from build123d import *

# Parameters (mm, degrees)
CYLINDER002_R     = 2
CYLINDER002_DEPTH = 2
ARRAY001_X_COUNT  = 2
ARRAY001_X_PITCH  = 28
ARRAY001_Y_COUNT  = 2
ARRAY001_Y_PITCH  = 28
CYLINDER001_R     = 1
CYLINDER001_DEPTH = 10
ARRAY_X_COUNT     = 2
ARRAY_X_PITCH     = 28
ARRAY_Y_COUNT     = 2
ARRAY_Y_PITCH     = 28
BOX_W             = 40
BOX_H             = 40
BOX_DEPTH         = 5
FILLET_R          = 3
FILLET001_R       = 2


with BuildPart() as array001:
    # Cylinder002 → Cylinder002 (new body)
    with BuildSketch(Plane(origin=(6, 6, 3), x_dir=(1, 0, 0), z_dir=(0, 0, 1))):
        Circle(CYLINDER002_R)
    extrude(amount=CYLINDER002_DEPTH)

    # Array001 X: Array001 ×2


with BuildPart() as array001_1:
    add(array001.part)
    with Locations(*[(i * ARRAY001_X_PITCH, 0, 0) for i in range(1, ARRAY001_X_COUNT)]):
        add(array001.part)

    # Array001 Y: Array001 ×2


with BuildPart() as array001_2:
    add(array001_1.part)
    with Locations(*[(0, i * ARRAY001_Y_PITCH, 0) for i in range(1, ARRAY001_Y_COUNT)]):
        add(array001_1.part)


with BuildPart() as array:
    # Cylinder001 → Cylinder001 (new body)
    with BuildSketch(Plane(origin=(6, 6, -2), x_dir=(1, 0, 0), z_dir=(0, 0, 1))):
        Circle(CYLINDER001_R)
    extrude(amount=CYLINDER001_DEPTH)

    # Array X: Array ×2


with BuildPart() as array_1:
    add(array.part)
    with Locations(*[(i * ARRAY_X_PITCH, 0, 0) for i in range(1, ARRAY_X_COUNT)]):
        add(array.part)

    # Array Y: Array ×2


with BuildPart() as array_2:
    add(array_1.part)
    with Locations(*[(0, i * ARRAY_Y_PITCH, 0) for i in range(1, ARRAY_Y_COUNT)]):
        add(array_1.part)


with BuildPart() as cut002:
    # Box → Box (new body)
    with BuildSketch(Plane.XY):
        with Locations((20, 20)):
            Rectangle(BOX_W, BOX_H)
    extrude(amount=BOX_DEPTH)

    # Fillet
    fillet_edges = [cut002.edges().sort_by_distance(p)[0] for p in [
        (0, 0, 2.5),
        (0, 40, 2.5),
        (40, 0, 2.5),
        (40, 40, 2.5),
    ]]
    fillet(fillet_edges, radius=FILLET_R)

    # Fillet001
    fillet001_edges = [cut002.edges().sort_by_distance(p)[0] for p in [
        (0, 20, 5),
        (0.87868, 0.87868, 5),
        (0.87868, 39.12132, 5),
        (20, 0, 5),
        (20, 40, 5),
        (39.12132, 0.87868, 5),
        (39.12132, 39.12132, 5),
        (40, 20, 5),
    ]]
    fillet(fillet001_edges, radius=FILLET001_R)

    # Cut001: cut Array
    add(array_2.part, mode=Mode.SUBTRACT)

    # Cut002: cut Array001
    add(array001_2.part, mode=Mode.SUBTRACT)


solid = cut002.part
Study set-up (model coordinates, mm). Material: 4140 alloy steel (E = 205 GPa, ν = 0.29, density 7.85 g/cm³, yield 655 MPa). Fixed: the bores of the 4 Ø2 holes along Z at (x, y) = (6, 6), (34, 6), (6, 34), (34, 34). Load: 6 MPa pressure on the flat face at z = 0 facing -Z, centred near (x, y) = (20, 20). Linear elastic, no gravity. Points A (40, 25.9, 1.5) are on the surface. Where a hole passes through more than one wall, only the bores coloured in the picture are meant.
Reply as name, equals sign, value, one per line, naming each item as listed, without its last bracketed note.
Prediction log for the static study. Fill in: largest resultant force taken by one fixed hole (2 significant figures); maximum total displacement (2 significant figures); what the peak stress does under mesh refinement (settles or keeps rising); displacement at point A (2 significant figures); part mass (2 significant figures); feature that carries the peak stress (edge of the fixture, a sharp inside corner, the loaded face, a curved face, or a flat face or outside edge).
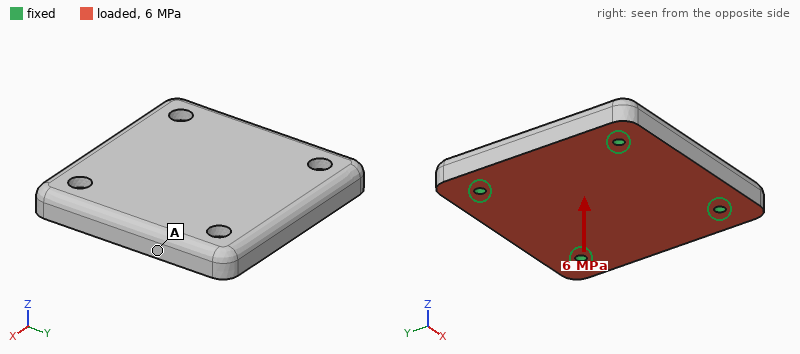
largest resultant force taken by one fixed hole = 2.5 kN
maximum total displacement = 21 µm
what the peak stress does under mesh refinement = keeps rising
displacement at point A = 7.7 µm
part mass = 60 g
feature that carries the peak stress = edge of the fixture
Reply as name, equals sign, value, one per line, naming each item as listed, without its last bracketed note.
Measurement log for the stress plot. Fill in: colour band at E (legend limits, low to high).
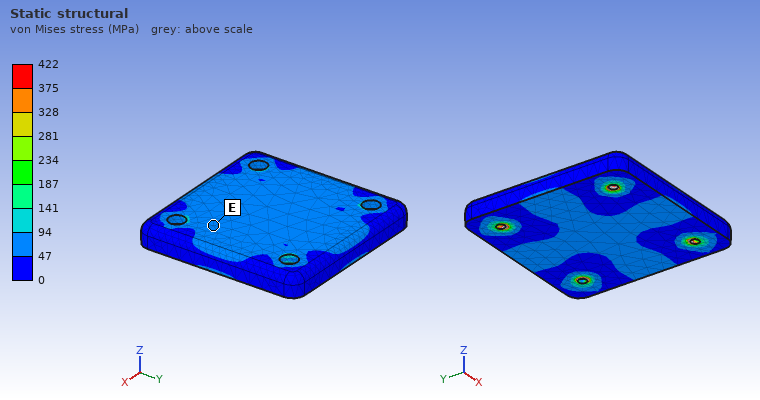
colour band at E = 47 to 94 MPa
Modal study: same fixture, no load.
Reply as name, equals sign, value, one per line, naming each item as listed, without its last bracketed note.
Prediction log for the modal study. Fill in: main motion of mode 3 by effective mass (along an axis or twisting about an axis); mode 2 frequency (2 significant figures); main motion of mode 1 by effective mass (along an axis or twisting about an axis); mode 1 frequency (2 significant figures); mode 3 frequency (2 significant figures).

main motion of mode 3 by effective mass = twisting about Y
mode 2 frequency = 21 kHz
main motion of mode 1 by effective mass = along Z
mode 1 frequency = 16 kHz
mode 3 frequency = 23 kHz
